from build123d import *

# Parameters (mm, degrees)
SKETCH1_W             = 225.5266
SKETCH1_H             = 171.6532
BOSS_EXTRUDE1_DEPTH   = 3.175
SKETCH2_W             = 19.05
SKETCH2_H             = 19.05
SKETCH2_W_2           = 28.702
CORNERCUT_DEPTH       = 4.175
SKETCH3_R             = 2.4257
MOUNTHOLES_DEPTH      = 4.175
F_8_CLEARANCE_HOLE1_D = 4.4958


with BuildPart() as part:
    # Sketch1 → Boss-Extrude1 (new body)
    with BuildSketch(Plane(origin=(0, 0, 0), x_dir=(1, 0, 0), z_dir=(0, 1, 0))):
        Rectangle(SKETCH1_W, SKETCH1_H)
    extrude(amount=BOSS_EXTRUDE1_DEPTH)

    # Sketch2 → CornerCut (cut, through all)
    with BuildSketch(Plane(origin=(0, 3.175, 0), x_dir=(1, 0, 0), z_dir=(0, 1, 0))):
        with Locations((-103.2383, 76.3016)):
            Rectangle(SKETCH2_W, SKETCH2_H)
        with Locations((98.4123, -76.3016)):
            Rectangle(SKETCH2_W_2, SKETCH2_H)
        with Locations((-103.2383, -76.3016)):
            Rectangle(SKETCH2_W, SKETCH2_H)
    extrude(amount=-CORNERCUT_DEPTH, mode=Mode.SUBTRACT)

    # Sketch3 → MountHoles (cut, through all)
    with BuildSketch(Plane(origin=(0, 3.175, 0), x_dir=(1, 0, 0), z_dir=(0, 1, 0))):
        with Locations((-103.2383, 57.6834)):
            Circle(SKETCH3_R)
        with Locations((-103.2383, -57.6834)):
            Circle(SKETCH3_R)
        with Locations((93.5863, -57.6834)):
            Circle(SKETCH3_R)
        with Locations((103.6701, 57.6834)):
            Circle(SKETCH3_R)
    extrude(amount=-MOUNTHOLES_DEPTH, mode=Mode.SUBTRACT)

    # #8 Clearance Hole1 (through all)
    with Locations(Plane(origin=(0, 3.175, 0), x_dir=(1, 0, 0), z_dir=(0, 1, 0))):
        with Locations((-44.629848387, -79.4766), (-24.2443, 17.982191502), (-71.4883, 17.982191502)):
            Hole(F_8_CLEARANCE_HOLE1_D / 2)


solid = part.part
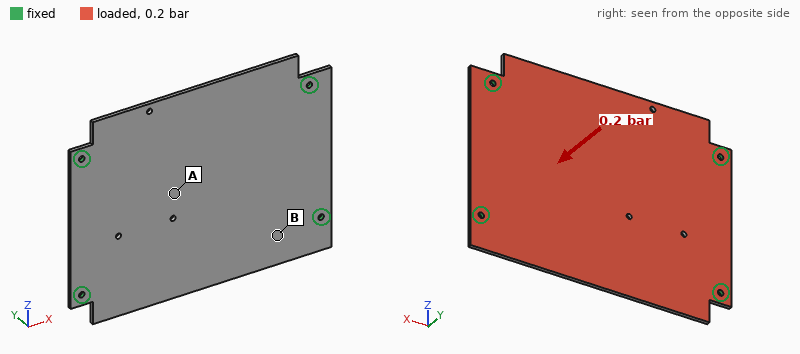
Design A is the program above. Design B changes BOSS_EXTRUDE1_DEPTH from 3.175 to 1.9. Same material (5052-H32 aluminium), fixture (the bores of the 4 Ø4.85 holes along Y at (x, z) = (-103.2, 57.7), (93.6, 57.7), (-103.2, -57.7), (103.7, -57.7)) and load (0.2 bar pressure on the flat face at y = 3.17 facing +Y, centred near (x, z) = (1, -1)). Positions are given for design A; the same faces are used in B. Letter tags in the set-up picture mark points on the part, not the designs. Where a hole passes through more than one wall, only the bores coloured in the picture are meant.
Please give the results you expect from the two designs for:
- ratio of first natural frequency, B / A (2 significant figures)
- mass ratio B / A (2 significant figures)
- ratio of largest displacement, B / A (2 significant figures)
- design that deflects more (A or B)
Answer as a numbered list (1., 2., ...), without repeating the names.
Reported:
1. 0.61
2. 0.60
3. 4.5
4. B
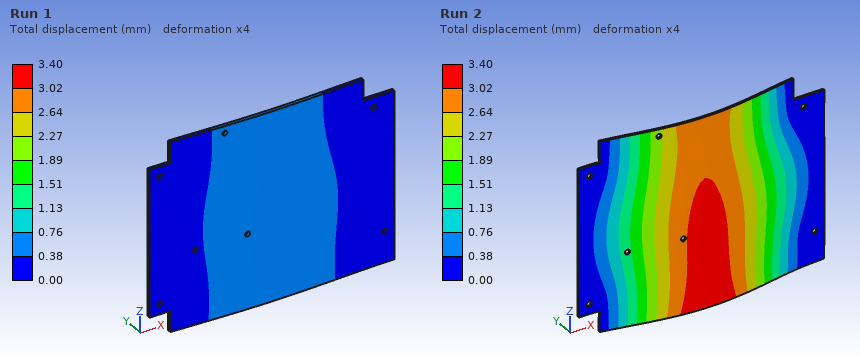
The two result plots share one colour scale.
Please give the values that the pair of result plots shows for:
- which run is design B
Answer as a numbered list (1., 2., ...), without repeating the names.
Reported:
1. Run 2
